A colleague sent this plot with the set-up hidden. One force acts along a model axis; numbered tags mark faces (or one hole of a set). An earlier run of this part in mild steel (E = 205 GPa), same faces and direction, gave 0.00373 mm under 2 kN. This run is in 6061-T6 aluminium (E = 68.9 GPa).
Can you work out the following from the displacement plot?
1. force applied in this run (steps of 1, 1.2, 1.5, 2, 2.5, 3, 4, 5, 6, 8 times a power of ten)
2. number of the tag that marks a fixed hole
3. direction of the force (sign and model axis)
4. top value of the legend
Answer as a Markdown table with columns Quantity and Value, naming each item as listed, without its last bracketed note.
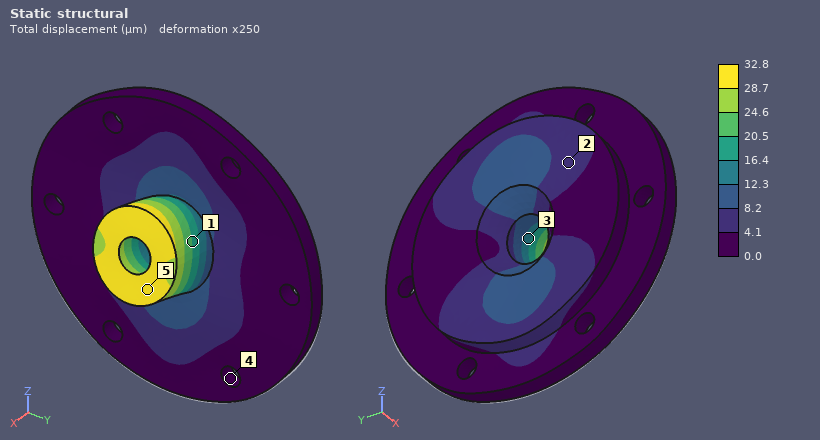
| Quantity | Value |
|---|---|
| force applied in this run | 6 kN |
| number of the tag that marks a fixed hole | 4 |
| direction of the force | +Z |
| top value of the legend | 32.8 µm |
